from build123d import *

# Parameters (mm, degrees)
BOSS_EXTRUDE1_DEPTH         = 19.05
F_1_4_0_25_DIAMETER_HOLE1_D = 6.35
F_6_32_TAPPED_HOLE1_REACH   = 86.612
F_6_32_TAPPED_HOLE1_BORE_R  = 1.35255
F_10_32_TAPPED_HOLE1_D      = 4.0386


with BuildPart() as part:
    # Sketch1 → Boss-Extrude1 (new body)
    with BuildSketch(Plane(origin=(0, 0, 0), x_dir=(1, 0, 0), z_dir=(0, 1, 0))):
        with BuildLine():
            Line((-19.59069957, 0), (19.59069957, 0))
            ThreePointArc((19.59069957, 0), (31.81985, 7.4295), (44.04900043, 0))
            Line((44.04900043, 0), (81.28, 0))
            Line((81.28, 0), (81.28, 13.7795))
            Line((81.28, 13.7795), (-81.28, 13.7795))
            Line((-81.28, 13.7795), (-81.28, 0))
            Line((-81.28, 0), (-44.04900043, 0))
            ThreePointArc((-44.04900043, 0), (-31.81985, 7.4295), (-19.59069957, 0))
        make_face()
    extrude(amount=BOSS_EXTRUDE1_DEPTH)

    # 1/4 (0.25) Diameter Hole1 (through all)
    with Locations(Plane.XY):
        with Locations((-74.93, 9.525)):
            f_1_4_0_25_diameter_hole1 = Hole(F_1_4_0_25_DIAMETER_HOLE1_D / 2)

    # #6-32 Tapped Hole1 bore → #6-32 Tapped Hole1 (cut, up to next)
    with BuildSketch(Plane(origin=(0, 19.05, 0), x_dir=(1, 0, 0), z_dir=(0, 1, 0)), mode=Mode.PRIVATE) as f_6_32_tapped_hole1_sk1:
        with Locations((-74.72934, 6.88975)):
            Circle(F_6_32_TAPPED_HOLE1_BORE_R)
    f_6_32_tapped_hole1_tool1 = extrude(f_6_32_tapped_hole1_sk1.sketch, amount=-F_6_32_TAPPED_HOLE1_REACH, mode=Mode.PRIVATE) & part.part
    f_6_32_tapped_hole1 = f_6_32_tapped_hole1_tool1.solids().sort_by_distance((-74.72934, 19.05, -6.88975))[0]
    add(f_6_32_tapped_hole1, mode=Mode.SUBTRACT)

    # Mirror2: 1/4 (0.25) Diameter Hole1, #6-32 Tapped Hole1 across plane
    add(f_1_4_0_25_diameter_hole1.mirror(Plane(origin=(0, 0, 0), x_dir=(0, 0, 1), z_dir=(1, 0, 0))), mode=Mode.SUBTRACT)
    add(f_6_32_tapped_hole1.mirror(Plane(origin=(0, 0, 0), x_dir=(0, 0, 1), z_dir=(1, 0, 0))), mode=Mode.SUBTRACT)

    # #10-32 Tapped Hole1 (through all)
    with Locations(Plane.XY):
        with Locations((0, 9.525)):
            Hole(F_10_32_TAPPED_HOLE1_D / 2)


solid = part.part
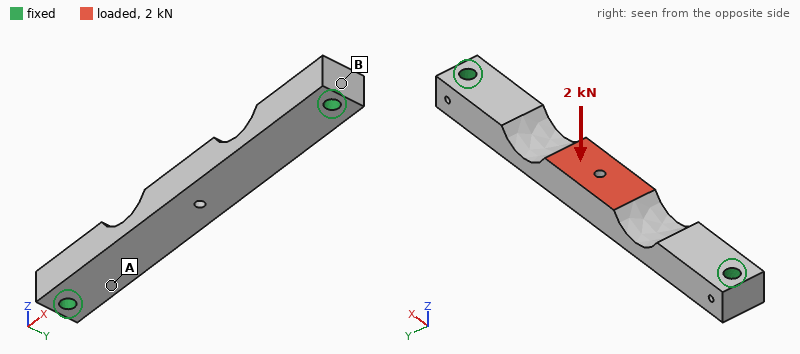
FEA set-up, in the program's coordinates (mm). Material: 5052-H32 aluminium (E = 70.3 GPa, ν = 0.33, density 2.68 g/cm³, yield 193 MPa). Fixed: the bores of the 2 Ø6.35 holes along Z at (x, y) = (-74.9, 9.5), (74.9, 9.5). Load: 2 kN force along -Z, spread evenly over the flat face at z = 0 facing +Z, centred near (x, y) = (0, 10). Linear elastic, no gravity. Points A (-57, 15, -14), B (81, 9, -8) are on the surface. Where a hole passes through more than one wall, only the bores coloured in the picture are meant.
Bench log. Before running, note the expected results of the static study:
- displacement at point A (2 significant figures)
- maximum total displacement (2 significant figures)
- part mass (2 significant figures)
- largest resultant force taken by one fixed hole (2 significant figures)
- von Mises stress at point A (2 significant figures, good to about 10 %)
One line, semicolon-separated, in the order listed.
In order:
0.024 mm; 0.14 mm; 98 g; 1.1 kN; 33 MPa
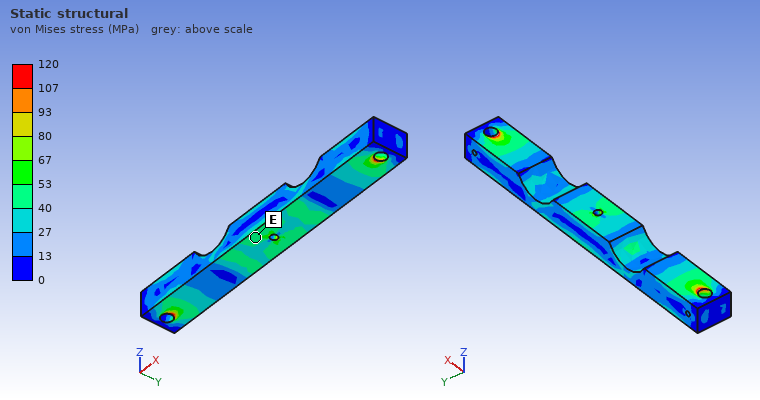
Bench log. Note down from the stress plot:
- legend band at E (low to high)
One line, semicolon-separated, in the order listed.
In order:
40 to 53 MPa
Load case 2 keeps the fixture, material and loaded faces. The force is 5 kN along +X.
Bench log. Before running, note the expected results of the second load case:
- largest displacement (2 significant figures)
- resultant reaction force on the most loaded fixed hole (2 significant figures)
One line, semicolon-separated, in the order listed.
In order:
58 µm; 2.6 kN
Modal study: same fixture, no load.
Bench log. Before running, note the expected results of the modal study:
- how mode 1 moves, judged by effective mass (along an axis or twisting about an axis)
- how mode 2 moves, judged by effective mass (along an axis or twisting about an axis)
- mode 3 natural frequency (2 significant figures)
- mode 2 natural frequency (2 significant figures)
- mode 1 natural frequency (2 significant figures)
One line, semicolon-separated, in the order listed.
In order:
along Z; along Y; 6100 Hz; 3500 Hz; 3100 Hz
